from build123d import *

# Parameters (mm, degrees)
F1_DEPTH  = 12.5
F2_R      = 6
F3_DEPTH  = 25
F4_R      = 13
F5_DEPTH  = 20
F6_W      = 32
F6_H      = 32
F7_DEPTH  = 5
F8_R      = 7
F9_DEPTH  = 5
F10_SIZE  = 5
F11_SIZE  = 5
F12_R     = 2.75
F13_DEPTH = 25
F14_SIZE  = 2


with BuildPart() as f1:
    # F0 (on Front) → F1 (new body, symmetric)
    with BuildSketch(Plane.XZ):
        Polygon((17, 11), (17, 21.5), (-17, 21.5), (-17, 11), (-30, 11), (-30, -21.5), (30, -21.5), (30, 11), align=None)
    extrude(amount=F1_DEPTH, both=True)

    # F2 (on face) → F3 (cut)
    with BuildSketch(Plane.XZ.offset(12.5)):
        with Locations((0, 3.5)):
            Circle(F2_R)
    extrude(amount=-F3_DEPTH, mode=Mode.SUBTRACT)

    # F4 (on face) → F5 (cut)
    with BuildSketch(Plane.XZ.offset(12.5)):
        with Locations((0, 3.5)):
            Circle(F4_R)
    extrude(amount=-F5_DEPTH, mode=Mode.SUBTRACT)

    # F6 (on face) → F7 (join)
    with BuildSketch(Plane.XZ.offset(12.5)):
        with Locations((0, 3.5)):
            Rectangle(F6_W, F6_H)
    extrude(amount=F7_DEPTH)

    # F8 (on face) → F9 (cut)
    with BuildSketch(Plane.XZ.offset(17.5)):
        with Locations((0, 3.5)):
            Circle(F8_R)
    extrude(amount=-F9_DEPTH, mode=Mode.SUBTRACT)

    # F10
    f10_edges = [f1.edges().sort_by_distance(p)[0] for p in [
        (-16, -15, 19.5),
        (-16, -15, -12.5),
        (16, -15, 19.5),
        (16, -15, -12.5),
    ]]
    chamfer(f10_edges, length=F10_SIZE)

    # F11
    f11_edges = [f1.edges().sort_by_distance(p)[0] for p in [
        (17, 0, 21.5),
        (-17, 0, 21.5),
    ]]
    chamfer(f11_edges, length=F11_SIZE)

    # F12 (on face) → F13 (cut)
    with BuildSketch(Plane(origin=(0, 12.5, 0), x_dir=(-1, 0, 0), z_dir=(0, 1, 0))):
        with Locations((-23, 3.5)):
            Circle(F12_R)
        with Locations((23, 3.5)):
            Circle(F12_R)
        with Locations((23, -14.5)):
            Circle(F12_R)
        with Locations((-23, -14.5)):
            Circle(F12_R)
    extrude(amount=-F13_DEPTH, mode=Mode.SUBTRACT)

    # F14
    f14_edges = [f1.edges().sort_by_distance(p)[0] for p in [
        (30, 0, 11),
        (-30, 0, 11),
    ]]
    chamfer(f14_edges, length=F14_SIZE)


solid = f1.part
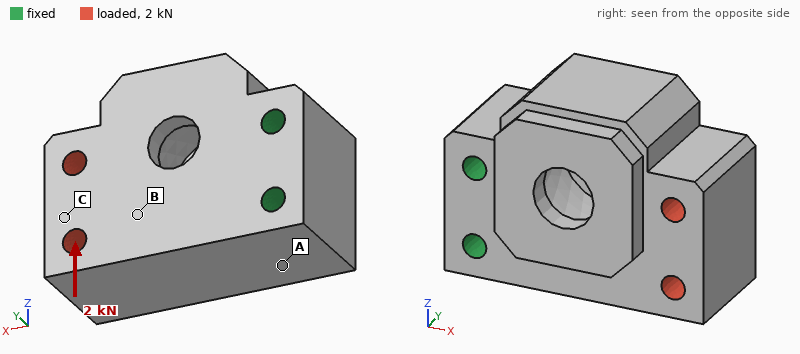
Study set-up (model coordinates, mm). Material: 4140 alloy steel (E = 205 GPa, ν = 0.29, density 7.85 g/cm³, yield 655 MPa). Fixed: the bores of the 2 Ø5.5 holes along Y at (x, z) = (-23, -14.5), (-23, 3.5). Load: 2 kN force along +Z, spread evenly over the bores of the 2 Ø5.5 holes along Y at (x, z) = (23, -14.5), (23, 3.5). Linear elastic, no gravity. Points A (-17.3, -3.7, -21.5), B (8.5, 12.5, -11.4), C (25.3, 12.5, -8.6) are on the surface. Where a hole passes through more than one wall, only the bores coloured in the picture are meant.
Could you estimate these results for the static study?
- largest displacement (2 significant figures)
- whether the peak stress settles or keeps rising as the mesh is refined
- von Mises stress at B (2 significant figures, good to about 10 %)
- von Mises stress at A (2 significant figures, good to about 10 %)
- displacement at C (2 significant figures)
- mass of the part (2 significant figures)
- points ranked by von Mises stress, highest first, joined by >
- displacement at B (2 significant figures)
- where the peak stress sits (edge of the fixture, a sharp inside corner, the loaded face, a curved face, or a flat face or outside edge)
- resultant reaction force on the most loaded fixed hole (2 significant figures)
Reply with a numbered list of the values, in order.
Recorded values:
1. 11 µm
2. keeps rising
3. 9.3 MPa
4. 17 MPa
5. 10.0 µm
6. 370 g
7. A > B > C
8. 5.8 µm
9. a sharp inside corner
10. 4.2 kN
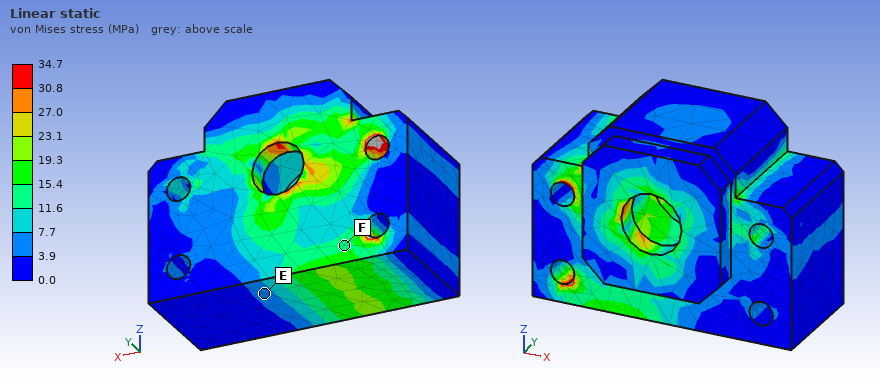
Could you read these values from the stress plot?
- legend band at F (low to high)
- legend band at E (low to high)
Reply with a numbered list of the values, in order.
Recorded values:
1. 11.6 to 15.4 MPa
2. 3.9 to 7.7 MPa
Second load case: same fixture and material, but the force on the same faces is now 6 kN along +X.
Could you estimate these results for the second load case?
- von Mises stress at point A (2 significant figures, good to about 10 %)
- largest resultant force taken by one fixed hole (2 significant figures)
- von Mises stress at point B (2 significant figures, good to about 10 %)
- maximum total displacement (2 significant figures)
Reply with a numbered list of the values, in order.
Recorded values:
1. 5.2 MPa
2. 3.1 kN
3. 13 MPa
4. 4.9 µm
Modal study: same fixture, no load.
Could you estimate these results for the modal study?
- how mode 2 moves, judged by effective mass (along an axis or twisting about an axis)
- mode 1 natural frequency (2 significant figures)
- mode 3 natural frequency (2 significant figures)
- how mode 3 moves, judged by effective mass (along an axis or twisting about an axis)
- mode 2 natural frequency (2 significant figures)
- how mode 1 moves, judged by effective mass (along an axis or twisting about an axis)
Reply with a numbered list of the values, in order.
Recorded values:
1. along Z
2. 5700 Hz
3. 12 kHz
4. twisting about X
5. 5900 Hz
6. along Y
